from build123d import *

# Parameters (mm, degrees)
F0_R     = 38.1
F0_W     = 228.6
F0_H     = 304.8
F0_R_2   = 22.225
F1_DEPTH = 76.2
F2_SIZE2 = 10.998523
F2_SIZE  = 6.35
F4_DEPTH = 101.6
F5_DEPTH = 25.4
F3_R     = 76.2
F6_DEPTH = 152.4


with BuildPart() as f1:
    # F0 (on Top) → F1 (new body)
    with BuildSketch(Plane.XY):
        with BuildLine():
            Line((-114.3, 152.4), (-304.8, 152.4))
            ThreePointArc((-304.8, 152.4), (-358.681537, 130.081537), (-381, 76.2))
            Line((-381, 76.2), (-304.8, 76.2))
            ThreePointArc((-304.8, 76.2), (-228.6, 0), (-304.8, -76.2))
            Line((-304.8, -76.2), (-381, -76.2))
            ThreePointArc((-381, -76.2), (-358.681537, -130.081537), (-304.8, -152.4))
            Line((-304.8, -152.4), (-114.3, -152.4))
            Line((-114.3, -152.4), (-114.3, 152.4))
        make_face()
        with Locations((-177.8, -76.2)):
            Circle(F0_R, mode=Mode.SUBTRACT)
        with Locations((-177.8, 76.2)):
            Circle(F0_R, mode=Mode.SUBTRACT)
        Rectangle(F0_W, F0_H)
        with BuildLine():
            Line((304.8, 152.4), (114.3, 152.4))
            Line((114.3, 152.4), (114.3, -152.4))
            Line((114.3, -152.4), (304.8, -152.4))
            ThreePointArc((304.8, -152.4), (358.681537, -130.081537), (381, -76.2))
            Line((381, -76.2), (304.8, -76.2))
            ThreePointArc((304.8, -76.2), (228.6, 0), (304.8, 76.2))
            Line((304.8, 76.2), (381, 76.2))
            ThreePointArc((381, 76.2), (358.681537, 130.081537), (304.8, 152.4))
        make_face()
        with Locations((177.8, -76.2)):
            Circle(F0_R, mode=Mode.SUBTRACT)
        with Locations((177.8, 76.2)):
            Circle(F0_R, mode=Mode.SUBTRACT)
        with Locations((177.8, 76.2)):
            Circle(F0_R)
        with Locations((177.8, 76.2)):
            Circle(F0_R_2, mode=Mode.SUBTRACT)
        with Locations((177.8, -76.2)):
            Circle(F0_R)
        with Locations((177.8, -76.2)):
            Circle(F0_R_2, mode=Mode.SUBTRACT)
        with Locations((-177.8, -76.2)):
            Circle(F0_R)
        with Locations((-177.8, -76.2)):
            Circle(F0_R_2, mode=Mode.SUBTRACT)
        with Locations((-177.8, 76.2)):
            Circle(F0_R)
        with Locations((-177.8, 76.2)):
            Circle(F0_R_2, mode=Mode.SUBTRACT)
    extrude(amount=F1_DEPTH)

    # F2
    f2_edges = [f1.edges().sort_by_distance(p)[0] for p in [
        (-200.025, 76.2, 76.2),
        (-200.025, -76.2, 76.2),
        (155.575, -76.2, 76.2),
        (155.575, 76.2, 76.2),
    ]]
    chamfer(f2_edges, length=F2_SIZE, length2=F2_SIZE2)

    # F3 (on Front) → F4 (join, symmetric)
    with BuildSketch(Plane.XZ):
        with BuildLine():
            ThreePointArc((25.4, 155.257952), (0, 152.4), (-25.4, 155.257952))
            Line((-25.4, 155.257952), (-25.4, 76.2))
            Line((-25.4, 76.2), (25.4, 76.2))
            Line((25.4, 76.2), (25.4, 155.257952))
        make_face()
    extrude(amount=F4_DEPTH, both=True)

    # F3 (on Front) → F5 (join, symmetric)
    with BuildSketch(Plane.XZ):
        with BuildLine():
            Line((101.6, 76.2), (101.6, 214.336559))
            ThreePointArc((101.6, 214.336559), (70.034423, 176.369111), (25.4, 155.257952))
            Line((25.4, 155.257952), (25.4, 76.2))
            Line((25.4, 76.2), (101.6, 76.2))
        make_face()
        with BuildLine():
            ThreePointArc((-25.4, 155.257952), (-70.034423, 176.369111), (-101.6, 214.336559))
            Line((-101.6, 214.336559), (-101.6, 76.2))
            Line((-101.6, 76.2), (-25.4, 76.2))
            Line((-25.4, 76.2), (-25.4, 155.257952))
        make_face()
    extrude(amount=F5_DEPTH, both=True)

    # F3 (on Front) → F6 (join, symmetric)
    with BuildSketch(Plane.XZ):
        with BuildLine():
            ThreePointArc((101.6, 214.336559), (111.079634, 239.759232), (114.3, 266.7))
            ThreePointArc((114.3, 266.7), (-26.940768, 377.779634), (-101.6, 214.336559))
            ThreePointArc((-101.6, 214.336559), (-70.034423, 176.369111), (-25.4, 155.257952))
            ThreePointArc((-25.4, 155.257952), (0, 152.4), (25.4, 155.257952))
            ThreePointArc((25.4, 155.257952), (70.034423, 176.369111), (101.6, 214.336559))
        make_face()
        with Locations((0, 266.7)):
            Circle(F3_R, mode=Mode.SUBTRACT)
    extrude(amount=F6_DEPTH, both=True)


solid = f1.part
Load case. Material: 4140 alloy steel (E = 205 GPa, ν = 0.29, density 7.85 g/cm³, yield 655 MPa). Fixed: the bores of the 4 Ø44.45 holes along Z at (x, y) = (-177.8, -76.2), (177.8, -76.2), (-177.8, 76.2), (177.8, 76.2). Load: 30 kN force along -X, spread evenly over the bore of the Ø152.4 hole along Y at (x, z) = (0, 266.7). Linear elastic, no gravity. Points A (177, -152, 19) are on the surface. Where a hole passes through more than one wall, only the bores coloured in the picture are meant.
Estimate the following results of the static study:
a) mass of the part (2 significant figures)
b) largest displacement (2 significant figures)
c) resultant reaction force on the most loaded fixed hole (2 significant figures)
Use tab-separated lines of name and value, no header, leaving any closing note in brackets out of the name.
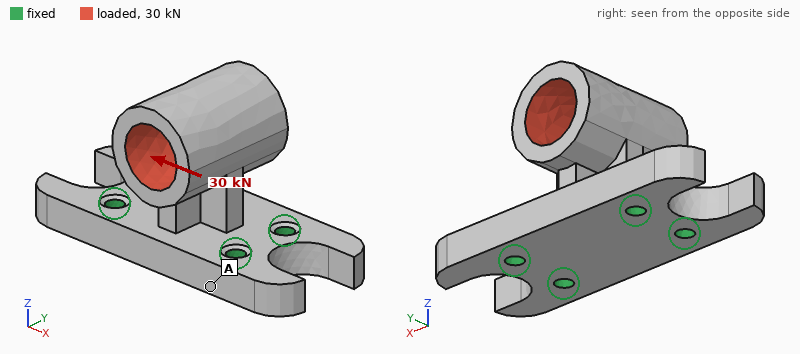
mass of the part	170 kg
largest displacement	49 µm
resultant reaction force on the most loaded fixed hole	15 kN
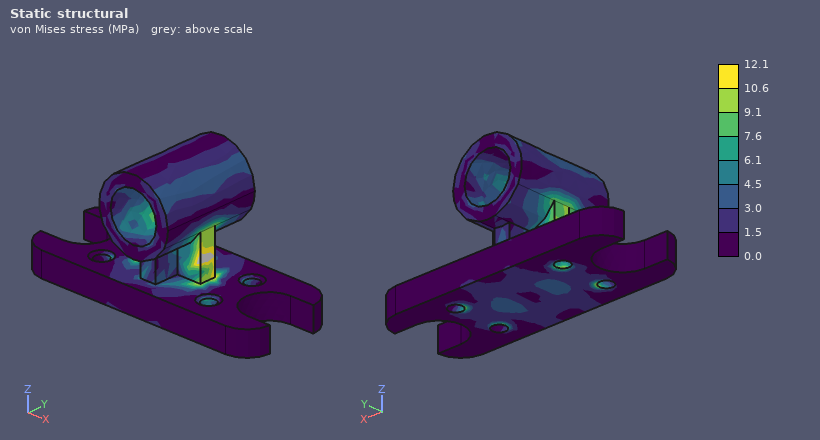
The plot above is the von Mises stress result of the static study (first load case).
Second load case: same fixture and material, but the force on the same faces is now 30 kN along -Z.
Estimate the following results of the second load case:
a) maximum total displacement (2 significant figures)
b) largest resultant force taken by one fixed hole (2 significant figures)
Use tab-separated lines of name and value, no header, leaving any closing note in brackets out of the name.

maximum total displacement	7.4 µm
largest resultant force taken by one fixed hole	7.7 kN
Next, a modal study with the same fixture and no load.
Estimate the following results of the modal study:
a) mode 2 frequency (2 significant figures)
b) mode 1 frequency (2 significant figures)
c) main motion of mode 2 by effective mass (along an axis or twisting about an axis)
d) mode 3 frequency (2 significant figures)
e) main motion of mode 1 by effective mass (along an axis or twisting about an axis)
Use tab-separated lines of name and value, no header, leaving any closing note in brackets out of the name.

mode 2 frequency	600 Hz
mode 1 frequency	520 Hz
main motion of mode 2 by effective mass	along X
mode 3 frequency	910 Hz
main motion of mode 1 by effective mass	along Y
